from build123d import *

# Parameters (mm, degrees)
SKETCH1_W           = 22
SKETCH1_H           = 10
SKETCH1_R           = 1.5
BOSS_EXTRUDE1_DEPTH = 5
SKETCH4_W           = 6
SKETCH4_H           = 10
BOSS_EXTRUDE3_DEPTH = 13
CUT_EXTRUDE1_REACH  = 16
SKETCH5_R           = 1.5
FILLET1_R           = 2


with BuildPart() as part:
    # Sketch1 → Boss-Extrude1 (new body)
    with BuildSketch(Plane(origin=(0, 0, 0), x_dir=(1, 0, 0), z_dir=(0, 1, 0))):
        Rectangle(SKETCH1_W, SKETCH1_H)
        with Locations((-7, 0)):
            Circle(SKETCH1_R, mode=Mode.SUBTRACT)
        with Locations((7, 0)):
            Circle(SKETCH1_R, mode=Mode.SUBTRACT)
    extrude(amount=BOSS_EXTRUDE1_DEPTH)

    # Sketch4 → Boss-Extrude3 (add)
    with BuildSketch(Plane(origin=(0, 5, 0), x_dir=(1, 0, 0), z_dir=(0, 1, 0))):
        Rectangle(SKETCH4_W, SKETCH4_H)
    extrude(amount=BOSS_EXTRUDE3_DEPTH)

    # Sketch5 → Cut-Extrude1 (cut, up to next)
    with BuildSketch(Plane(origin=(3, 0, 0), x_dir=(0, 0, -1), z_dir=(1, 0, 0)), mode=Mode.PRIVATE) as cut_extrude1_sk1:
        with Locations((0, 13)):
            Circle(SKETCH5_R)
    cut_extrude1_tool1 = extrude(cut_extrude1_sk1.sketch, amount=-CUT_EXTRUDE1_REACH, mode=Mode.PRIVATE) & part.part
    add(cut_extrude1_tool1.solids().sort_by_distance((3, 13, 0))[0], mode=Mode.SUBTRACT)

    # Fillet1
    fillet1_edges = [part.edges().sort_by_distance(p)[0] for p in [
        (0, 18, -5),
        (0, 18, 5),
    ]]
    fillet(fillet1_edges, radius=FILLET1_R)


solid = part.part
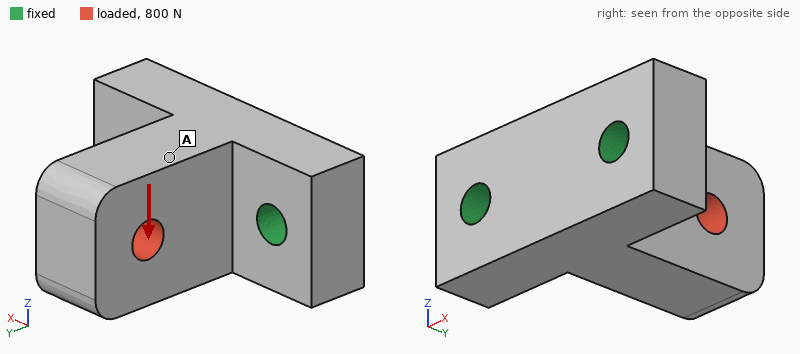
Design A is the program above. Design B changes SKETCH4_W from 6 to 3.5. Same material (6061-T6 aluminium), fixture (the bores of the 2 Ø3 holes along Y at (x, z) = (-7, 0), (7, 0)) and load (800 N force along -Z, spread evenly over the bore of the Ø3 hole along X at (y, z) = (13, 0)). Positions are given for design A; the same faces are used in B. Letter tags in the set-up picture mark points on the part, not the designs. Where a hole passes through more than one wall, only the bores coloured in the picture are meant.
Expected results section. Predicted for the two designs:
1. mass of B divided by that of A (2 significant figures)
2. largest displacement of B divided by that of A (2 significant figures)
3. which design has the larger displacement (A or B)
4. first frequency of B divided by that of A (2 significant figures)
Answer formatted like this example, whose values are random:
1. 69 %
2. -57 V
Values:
1. 0.83
2. 1.4
3. B
4. 0.82
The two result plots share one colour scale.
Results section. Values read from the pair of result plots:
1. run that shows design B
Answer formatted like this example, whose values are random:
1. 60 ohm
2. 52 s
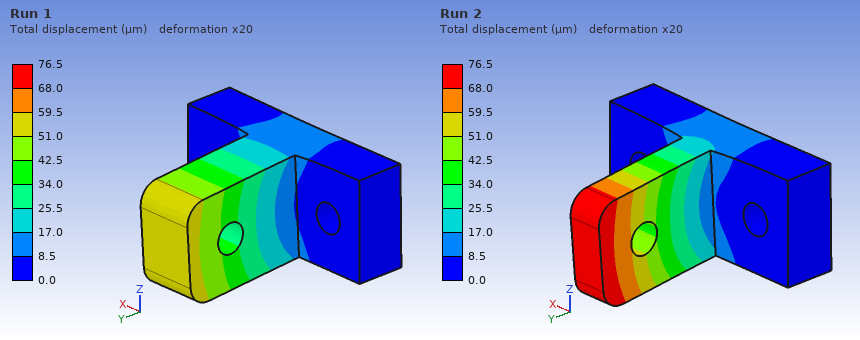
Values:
1. Run 2
